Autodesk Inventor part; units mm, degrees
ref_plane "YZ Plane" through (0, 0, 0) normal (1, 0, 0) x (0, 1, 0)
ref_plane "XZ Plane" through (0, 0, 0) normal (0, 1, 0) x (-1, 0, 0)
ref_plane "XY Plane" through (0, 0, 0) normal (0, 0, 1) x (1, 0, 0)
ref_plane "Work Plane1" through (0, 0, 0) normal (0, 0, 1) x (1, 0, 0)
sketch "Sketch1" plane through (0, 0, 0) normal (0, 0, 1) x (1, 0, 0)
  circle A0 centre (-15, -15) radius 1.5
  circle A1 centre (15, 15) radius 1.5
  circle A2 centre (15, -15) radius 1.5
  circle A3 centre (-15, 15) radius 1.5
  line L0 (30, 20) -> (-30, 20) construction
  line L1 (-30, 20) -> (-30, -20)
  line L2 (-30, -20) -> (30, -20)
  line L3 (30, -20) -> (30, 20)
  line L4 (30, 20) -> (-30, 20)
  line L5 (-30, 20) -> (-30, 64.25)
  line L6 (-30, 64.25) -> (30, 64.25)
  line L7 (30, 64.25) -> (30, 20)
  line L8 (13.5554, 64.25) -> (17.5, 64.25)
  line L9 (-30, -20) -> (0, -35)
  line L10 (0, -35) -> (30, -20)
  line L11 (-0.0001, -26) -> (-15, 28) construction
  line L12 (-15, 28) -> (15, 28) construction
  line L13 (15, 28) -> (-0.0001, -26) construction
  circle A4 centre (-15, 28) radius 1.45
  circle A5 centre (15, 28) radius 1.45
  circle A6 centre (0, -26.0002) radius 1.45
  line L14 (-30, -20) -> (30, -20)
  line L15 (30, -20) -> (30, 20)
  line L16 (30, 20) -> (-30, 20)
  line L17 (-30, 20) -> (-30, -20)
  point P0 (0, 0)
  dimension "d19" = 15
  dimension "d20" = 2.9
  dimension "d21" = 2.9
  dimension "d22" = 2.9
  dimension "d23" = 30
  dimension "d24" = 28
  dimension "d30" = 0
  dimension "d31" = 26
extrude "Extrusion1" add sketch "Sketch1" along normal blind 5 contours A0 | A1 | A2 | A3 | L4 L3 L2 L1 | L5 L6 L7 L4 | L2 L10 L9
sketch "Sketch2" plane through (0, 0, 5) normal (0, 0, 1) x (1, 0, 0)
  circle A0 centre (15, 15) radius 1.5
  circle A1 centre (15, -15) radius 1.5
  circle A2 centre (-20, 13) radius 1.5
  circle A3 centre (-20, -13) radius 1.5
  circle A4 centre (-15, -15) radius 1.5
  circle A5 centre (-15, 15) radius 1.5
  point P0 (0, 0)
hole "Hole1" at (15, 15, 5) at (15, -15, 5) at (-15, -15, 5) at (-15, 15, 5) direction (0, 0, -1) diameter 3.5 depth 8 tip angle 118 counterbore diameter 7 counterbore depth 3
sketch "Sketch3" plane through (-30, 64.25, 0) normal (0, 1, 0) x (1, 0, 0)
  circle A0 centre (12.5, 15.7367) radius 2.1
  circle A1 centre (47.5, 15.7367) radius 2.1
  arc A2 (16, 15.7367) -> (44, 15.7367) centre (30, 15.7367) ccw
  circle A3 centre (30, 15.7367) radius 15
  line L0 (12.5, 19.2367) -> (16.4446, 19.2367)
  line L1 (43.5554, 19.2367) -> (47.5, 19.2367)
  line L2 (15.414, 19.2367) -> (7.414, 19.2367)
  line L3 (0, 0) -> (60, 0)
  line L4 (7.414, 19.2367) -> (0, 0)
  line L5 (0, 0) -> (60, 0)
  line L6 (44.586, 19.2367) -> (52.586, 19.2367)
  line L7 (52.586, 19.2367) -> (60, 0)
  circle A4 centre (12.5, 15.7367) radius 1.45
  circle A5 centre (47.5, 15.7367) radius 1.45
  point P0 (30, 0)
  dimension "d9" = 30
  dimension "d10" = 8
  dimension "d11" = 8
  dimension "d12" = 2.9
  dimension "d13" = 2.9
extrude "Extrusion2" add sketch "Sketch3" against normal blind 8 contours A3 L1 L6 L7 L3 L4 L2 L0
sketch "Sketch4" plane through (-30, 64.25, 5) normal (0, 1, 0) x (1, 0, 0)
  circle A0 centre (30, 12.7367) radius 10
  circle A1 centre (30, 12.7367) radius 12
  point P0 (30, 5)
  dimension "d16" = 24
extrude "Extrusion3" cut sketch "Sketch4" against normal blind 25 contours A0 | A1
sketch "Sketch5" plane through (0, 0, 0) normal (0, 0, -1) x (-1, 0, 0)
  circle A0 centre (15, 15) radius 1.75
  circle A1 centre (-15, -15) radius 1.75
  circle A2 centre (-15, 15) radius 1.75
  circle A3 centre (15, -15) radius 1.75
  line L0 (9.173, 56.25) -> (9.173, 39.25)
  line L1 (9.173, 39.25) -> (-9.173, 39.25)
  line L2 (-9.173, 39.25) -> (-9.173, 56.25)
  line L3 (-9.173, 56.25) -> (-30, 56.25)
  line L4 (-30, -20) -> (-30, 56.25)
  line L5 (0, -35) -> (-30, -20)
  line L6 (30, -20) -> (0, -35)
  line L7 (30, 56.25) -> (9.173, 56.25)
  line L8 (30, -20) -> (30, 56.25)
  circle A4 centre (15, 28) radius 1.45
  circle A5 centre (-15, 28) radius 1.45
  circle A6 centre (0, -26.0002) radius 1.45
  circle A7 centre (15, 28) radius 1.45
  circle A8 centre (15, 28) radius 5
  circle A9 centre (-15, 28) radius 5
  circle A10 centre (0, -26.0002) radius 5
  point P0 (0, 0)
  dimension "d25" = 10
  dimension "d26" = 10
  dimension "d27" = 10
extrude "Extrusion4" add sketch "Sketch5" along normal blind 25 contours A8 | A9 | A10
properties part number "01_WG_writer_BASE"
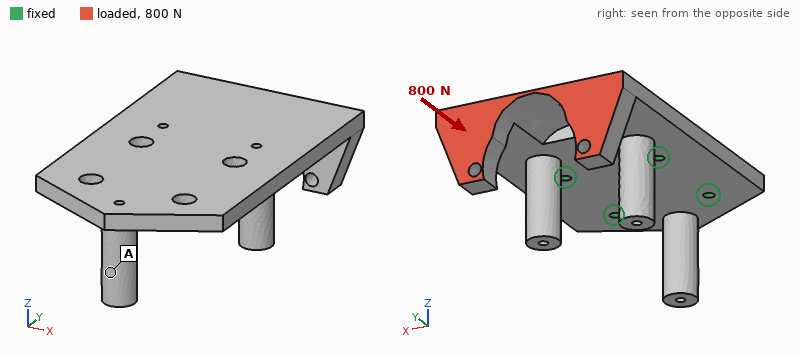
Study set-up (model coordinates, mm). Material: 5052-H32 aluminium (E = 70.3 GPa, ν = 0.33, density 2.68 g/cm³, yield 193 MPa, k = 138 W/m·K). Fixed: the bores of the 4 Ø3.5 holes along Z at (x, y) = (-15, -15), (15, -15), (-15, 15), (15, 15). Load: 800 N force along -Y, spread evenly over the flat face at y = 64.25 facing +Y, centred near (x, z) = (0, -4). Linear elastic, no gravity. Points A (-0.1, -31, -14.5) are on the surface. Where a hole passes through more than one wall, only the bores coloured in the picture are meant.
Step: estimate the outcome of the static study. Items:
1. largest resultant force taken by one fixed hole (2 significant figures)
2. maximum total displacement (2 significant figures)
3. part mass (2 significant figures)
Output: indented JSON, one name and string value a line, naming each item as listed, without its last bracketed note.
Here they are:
{
  "largest resultant force taken by one fixed hole": "480 N",
  "maximum total displacement": "0.22 mm",
  "part mass": "93 g"
}
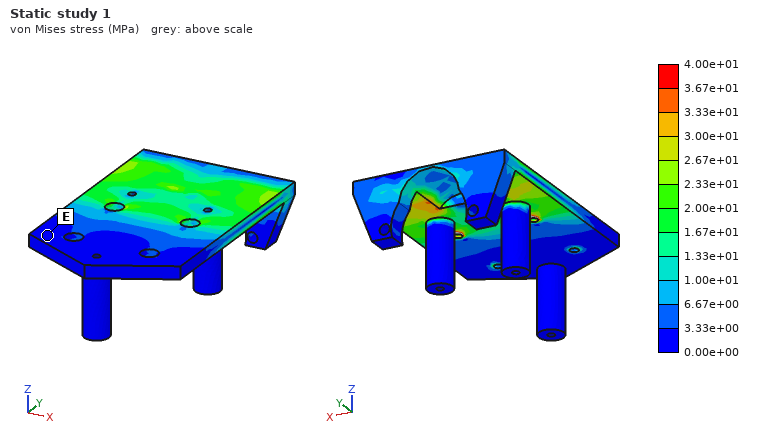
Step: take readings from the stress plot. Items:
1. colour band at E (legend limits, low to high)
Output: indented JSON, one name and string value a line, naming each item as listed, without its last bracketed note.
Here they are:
{
  "colour band at E": "0.00e+00 to 3.33e+00 MPa"
}
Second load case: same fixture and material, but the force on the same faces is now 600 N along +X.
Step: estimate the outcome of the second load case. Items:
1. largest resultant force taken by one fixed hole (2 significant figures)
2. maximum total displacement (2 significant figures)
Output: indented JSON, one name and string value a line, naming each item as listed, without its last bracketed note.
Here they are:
{
  "largest resultant force taken by one fixed hole": "610 N",
  "maximum total displacement": "0.10 mm"
}
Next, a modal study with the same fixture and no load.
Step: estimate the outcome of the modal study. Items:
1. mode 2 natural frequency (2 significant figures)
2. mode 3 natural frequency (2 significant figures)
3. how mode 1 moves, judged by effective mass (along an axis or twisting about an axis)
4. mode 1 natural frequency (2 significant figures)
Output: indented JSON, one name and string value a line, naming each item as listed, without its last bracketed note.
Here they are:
{
  "mode 2 natural frequency": "1800 Hz",
  "mode 3 natural frequency": "3600 Hz",
  "how mode 1 moves, judged by effective mass": "along Z",
  "mode 1 natural frequency": "1100 Hz"
}
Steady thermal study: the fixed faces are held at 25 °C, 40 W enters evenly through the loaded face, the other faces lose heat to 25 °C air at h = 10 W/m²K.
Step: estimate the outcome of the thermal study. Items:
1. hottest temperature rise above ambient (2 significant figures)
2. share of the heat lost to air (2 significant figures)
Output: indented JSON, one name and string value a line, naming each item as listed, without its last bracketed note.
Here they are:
{
  "hottest temperature rise above ambient": "61 K",
  "share of the heat lost to air": "8.6 %"
}
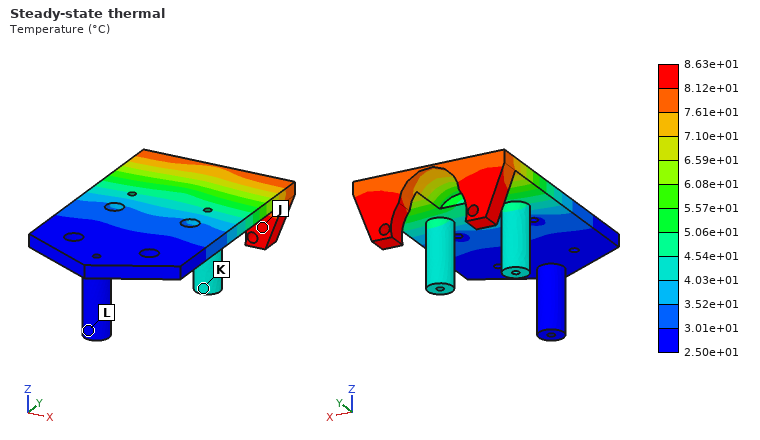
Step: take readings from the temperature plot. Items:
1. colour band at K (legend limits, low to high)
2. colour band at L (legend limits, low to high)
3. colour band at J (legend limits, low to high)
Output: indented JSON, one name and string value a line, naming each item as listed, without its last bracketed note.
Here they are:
{
  "colour band at K": "4.03e+01 to 4.54e+01 °C",
  "colour band at L": "2.50e+01 to 3.01e+01 °C",
  "colour band at J": "8.12e+01 to 8.63e+01 °C"
}
